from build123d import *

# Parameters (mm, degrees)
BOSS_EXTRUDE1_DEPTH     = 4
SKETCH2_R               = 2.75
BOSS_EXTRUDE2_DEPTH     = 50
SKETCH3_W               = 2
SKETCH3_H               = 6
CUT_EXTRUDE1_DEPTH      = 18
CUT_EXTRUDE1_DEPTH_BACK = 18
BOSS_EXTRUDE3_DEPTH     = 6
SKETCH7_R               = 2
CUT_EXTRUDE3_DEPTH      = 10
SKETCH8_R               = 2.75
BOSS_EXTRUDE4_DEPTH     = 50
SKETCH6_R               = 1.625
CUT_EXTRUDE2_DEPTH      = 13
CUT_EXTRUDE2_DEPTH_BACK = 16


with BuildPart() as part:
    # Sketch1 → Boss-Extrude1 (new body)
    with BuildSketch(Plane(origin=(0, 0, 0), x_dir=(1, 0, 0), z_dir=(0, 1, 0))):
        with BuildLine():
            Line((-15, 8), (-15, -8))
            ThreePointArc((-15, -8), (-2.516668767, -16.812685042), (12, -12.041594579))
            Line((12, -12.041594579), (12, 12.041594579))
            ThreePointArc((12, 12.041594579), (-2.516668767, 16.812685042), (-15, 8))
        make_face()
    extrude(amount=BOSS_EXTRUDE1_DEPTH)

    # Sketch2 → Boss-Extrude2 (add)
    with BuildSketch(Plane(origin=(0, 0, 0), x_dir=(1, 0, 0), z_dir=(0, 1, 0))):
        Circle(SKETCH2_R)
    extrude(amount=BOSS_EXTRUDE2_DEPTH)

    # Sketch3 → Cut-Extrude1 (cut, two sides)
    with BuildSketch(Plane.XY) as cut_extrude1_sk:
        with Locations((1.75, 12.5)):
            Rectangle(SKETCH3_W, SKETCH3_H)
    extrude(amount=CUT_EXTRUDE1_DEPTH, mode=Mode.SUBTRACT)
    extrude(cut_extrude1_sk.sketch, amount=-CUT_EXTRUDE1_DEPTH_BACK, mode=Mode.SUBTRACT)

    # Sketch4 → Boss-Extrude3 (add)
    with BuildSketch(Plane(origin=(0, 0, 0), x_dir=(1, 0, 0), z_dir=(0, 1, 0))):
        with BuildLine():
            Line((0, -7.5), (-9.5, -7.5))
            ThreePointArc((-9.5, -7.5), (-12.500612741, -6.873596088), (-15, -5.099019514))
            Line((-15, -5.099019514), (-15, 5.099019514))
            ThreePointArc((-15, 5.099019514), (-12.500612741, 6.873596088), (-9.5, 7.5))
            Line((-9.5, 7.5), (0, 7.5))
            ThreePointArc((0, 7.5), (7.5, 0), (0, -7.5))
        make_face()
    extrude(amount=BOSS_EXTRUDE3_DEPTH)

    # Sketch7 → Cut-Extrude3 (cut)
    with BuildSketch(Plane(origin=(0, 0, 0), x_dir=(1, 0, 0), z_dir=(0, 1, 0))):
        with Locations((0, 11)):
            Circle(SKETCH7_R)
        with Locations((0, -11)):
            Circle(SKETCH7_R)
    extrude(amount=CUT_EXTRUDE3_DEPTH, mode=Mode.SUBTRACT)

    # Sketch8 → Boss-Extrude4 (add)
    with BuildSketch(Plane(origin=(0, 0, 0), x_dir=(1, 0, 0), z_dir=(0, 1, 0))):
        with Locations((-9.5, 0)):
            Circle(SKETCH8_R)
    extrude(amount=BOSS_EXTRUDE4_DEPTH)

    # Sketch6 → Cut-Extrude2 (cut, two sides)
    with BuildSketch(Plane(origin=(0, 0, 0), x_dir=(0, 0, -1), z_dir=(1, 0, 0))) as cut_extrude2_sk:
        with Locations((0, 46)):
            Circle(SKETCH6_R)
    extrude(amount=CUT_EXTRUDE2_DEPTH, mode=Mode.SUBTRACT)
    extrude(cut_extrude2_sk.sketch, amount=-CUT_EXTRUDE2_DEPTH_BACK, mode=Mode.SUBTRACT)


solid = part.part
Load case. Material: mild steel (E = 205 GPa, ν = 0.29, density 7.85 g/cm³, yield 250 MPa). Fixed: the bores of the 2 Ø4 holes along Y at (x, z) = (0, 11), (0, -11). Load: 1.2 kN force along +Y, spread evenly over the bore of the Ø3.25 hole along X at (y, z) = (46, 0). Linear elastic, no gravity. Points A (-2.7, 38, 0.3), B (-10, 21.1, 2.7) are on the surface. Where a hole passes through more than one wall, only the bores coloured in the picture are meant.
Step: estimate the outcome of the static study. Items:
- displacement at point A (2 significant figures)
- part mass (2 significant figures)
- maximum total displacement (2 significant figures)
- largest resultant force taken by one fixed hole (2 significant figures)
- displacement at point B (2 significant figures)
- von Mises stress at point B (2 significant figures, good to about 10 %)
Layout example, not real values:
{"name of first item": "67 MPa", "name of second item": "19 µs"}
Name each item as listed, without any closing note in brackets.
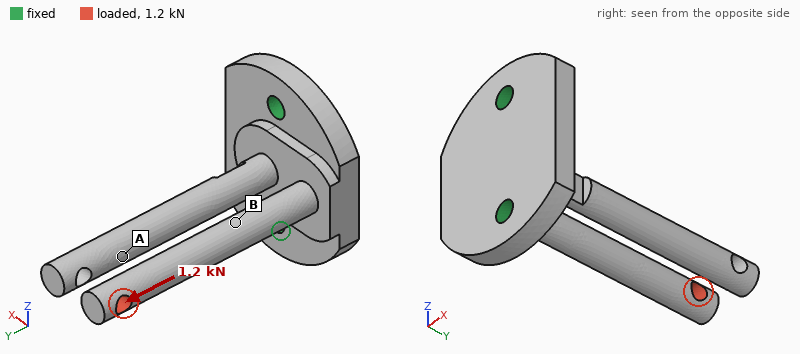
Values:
{"displacement at point A": "29 µm", "part mass": "45 g", "maximum total displacement": "67 µm", "largest resultant force taken by one fixed hole": "680 N", "displacement at point B": "29 µm", "von Mises stress at point B": "50 MPa"}
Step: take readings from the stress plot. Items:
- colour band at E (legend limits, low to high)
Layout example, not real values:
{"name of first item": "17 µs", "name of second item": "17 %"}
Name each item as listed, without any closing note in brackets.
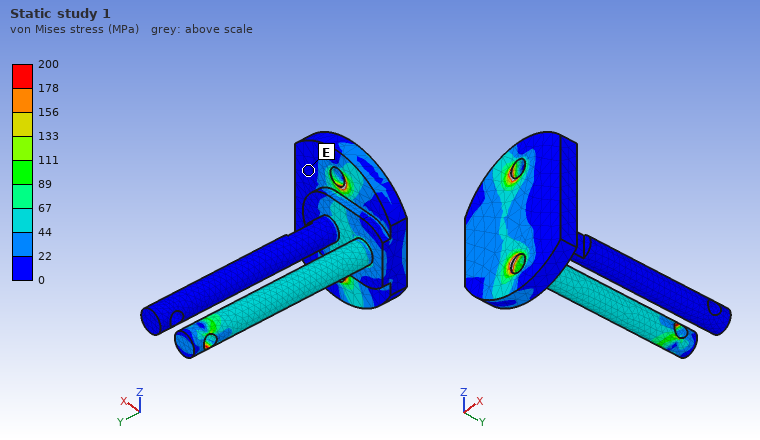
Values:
{"colour band at E": "0 to 22 MPa"}
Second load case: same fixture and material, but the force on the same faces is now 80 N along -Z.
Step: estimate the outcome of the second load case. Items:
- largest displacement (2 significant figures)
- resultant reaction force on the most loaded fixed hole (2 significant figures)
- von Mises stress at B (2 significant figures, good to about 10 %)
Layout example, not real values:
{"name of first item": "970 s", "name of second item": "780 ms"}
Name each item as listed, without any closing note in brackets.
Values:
{"largest displacement": "0.25 mm", "resultant reaction force on the most loaded fixed hole": "190 N", "von Mises stress at B": "120 MPa"}
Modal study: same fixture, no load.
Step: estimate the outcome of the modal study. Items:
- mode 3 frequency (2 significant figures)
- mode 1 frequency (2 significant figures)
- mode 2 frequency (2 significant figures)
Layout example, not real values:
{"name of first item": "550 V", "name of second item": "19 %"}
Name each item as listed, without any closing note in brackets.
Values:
{"mode 3 frequency": "1900 Hz", "mode 1 frequency": "1400 Hz", "mode 2 frequency": "1900 Hz"}
